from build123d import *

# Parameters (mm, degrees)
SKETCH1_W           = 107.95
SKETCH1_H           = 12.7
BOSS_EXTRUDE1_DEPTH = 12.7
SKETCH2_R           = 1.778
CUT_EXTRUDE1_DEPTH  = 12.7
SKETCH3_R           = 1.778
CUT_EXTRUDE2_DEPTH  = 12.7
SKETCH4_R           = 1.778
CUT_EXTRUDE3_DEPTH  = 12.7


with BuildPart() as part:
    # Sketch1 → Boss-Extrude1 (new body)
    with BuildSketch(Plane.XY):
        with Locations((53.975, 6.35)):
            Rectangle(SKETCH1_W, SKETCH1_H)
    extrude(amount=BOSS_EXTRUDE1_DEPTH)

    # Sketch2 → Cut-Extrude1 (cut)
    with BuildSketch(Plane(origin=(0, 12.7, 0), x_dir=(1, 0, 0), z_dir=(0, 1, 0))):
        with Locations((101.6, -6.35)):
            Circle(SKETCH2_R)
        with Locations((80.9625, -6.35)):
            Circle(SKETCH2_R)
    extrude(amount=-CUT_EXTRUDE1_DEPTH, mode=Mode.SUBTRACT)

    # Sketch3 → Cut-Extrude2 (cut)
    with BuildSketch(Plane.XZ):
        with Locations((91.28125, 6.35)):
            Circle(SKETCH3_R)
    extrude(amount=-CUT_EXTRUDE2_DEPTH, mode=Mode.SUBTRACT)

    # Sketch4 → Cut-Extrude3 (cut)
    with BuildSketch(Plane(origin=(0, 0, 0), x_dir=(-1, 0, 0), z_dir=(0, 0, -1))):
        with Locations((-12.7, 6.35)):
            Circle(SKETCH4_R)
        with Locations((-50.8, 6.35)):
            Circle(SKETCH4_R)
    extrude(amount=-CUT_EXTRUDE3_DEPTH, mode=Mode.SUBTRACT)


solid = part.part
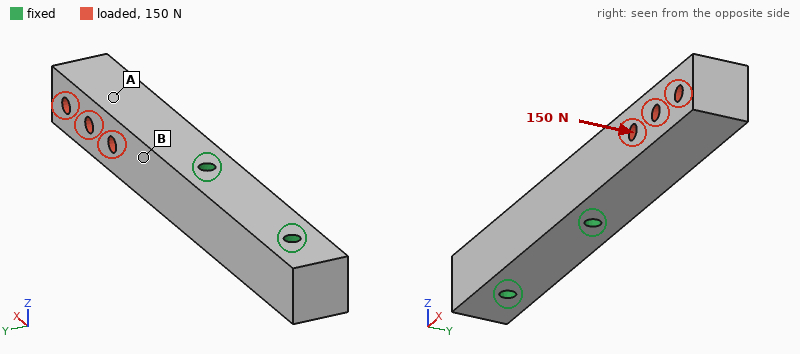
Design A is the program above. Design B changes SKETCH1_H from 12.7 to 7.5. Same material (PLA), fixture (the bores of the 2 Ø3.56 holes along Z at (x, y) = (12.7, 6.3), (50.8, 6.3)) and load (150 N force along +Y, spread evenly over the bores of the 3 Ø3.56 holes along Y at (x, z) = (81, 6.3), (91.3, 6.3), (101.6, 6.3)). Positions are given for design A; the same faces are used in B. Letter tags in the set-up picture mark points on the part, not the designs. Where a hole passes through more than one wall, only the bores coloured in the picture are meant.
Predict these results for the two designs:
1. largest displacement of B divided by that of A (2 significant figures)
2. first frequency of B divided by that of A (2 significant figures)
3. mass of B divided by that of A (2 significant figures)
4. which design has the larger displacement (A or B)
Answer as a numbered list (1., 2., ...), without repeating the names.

1. 3.7
2. 0.69
3. 0.58
4. B
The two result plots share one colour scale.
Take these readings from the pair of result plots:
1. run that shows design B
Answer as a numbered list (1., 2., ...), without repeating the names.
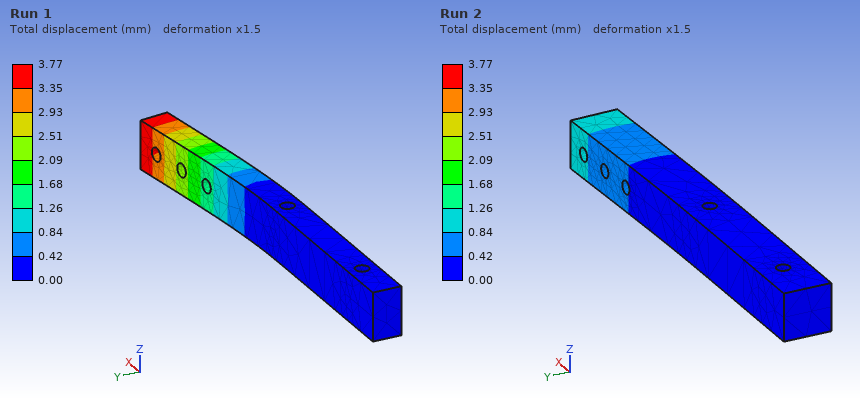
1. Run 1
